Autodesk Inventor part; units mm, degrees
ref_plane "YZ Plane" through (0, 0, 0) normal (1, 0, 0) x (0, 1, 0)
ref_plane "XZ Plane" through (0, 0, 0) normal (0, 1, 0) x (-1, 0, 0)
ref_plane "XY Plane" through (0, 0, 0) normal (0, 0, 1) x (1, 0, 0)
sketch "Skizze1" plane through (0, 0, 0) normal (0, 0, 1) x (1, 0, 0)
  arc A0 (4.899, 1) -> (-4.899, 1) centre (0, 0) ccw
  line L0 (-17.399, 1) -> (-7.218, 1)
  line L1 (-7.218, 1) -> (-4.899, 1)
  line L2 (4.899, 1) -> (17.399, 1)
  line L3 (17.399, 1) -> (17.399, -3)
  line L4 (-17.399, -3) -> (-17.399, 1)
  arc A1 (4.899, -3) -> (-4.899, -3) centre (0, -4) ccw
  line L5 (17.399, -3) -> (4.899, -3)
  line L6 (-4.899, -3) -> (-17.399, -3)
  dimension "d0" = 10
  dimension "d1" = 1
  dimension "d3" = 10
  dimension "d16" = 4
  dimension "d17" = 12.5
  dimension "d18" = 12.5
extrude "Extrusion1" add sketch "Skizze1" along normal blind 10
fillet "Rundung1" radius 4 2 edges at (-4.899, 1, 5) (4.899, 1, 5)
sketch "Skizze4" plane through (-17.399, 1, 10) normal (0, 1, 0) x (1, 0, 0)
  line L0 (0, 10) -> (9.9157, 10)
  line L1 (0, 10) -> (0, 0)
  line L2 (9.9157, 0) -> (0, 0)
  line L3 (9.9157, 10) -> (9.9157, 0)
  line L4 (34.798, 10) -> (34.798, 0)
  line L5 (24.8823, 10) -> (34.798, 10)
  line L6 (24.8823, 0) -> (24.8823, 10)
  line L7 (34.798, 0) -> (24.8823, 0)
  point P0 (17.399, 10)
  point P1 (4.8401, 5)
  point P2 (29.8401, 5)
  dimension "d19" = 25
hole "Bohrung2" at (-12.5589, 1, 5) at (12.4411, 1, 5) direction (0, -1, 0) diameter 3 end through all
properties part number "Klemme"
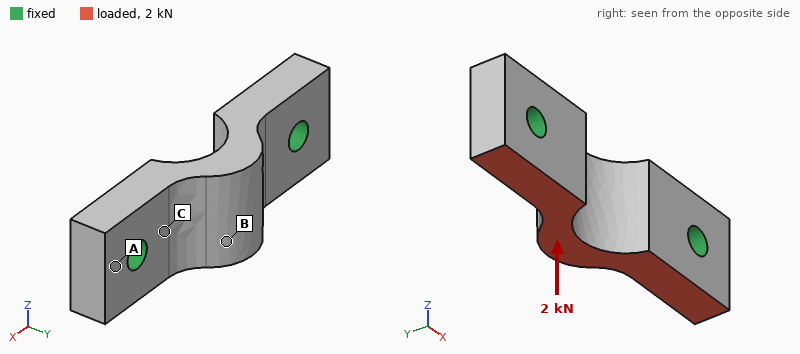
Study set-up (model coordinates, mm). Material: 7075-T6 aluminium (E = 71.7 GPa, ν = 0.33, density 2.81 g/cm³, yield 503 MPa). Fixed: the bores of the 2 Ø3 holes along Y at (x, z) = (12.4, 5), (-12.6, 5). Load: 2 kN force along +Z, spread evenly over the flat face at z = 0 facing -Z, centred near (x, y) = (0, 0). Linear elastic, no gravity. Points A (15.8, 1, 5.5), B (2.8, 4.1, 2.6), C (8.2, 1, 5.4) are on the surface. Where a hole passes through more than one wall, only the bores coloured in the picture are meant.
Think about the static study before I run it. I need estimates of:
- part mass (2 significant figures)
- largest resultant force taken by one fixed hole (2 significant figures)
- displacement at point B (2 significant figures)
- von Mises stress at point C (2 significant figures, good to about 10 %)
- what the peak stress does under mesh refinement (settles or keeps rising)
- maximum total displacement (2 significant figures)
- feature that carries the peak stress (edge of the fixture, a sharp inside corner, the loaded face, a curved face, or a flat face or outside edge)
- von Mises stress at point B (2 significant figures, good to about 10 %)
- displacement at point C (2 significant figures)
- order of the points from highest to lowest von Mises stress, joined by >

3.8 g
1.0 kN
22 µm
66 MPa
keeps rising
27 µm
edge of the fixture
26 MPa
6.6 µm
C > B > A
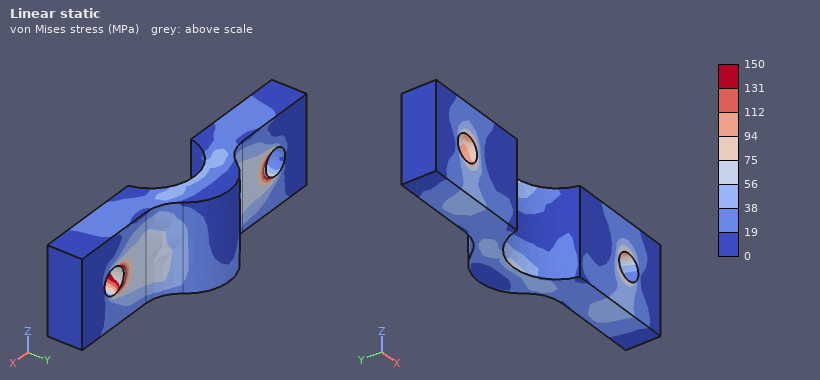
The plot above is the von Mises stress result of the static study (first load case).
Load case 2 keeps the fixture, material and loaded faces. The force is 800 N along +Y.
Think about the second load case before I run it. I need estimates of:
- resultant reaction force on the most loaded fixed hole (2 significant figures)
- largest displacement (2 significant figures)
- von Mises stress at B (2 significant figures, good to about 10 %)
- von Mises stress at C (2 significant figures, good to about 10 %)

430 N
20 µm
16 MPa
33 MPa
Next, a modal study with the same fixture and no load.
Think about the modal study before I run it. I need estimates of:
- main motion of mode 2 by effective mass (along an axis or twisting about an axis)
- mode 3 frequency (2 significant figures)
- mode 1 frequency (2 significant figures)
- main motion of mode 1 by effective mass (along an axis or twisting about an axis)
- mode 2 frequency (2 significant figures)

along Y
52 kHz
26 kHz
along Z
34 kHz
